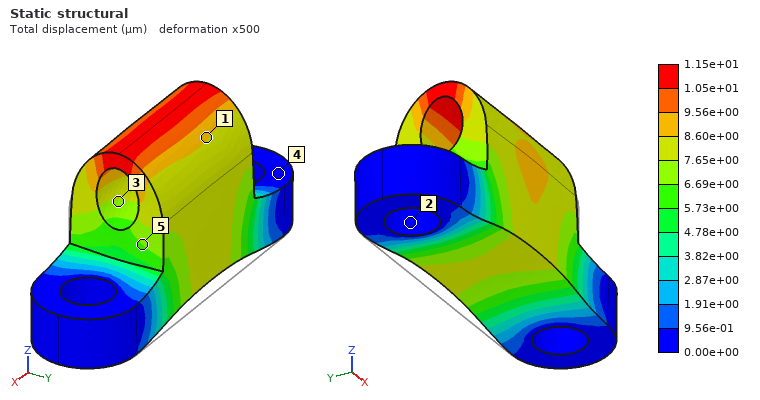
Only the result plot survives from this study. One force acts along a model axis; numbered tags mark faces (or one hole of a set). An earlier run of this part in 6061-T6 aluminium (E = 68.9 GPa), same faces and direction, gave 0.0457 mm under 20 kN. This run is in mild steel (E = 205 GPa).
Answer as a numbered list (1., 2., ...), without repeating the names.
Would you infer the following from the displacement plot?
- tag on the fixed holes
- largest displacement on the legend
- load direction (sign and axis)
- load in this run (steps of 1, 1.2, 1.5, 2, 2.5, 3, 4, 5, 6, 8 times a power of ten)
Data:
1. 2
2. 1.15e+01 µm
3. +Z
4. 15 kN
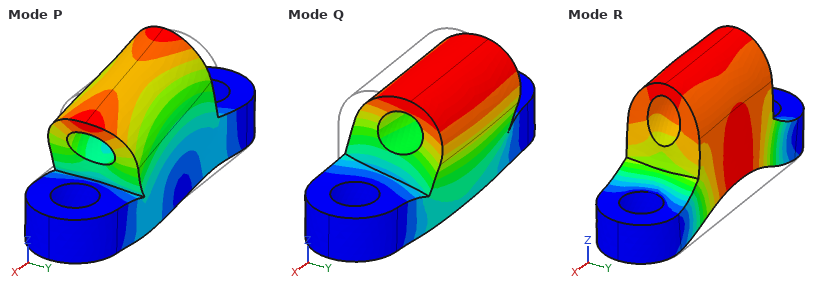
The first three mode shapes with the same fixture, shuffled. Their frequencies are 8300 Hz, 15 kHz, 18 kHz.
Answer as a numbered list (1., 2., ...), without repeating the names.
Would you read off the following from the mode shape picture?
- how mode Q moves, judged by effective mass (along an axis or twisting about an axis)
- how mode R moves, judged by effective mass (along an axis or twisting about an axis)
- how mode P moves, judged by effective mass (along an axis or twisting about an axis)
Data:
1. along Y
2. along Z
3. along X
